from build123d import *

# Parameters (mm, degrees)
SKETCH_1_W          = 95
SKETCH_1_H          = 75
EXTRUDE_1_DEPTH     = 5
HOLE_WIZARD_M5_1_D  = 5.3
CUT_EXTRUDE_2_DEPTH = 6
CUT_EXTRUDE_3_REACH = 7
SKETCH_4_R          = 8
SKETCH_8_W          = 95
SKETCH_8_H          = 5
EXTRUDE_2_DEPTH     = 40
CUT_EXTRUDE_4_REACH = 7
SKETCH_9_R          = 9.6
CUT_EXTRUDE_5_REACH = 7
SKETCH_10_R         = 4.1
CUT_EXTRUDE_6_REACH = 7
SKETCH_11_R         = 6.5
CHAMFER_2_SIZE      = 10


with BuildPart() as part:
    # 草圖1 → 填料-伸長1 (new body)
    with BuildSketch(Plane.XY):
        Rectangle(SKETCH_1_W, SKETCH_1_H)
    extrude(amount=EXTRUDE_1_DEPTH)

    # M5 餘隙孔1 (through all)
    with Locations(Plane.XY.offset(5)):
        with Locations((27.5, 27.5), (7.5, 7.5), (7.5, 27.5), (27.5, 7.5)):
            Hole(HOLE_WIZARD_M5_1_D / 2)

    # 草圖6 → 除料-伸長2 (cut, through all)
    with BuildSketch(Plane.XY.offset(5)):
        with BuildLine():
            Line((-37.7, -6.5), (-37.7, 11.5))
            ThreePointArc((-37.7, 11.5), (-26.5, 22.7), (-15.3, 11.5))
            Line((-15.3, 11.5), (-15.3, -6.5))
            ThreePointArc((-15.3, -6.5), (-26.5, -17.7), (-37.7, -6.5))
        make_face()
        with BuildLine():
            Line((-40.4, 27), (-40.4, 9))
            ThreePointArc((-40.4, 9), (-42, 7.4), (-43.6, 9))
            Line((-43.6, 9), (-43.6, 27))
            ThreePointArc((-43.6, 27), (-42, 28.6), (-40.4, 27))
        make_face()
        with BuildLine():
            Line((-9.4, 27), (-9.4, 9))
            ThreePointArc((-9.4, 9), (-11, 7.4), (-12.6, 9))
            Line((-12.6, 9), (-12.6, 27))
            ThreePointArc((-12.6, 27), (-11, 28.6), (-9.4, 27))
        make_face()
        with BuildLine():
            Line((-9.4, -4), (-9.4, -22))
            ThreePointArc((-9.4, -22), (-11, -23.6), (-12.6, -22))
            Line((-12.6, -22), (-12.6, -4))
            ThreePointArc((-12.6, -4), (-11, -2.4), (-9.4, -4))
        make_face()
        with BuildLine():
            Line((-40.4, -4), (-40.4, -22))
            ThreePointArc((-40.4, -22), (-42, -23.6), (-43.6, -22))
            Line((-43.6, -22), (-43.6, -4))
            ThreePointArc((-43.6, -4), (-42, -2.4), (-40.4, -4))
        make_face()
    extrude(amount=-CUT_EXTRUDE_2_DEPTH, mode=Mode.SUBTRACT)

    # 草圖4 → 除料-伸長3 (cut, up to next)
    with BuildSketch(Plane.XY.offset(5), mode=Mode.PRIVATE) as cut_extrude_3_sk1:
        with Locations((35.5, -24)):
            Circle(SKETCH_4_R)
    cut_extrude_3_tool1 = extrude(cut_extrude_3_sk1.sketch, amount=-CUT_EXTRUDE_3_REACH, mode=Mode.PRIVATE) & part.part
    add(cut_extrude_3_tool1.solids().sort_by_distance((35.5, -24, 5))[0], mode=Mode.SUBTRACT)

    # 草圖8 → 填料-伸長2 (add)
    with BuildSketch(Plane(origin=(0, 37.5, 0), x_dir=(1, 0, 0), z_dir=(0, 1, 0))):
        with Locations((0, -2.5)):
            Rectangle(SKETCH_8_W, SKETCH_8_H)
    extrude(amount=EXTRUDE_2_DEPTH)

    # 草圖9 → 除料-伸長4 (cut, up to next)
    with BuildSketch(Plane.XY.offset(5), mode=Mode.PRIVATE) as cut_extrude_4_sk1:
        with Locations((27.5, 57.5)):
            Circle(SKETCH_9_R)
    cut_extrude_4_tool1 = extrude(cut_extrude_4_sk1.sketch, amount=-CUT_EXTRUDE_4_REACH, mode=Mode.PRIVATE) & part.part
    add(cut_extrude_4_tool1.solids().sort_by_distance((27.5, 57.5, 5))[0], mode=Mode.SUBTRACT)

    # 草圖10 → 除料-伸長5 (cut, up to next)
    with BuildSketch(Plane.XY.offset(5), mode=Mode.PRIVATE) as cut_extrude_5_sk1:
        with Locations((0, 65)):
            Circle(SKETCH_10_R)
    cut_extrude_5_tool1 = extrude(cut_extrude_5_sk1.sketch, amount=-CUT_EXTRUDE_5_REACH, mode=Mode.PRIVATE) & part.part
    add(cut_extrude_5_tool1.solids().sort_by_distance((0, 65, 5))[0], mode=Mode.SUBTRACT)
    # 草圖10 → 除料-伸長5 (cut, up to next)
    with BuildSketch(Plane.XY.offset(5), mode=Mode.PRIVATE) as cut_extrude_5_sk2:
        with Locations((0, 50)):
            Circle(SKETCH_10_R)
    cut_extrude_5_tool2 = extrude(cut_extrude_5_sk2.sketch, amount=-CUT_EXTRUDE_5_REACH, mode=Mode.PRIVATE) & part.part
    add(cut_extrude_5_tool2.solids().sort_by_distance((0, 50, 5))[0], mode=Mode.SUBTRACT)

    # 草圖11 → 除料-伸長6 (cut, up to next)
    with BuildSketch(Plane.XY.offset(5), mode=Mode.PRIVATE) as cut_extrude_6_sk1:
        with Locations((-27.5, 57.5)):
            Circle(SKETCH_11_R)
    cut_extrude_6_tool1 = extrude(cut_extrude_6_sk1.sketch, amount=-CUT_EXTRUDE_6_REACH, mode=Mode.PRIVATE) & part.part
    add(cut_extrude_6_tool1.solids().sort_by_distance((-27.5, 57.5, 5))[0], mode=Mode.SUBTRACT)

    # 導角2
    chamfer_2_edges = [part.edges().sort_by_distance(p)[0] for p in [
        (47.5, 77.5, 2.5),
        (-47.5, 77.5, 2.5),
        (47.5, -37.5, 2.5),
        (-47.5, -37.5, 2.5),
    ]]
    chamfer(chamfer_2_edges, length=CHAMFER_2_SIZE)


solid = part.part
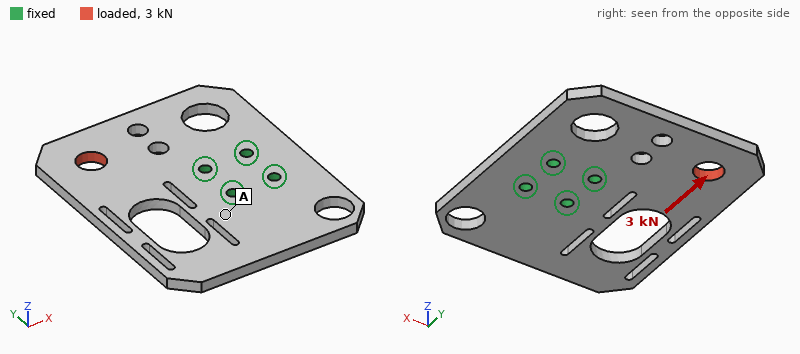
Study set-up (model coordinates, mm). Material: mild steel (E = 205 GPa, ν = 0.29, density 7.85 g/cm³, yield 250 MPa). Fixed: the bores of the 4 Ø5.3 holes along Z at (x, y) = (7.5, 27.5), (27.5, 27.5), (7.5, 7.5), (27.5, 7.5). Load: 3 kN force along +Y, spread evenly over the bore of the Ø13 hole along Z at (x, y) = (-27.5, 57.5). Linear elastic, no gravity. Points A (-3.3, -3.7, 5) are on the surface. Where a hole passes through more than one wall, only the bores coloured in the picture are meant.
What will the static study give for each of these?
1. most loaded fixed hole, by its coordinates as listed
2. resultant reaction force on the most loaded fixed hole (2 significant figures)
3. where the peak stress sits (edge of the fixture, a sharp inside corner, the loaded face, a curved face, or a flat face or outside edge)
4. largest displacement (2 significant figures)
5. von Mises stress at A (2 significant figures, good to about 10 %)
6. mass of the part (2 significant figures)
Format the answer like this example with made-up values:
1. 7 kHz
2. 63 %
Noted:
1. (7.5, 27.5)
2. 3.1 kN
3. a curved face
4. 27 µm
5. 14 MPa
6. 350 g
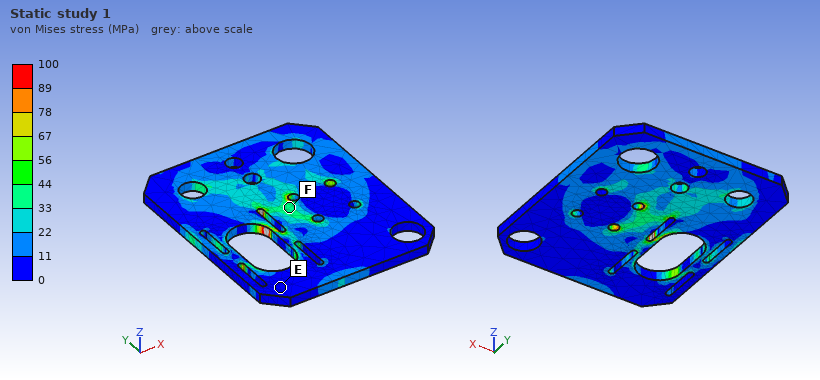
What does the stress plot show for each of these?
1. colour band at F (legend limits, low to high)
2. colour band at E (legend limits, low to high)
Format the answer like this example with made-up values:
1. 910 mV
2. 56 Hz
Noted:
1. 33 to 44 MPa
2. 0 to 11 MPa
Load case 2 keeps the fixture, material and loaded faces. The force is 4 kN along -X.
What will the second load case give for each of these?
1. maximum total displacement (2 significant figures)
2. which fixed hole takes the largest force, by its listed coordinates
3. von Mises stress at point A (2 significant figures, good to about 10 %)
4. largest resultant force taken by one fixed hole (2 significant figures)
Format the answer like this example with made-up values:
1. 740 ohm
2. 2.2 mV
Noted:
1. 27 µm
2. (7.5, 27.5)
3. 10 MPa
4. 3.7 kN
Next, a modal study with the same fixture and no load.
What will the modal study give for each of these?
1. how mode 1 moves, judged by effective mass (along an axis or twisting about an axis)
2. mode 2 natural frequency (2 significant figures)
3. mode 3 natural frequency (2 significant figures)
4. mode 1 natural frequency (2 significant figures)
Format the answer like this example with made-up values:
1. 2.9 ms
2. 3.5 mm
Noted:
1. along Z
2. 1200 Hz
3. 1800 Hz
4. 1000 Hz
